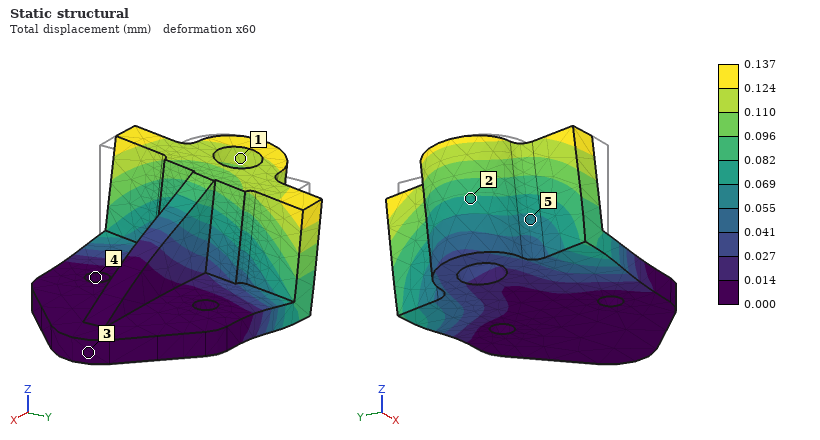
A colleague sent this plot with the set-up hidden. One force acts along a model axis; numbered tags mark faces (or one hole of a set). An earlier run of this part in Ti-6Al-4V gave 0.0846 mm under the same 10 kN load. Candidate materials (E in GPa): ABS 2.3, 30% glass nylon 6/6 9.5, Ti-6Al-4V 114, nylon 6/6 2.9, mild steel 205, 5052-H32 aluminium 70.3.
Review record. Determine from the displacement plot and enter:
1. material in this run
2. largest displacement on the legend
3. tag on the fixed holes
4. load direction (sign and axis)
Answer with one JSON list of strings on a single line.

["5052-H32 aluminium", "0.137 mm", "4", "+Y"]
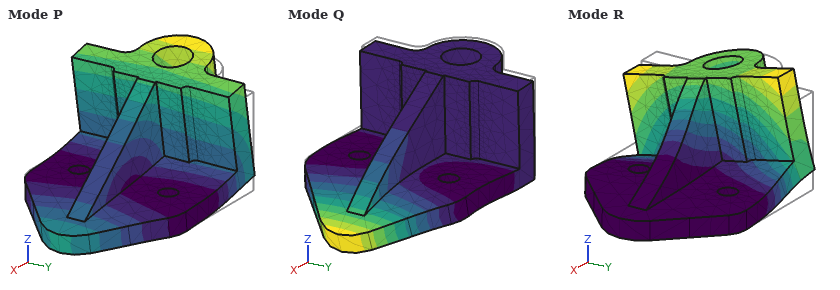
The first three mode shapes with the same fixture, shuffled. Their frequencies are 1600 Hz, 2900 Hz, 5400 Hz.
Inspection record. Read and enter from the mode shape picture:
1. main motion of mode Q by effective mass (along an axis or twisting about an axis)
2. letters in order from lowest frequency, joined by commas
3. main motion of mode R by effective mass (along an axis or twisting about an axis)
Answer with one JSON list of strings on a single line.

["along Z", "P, R, Q", "along Y"]
